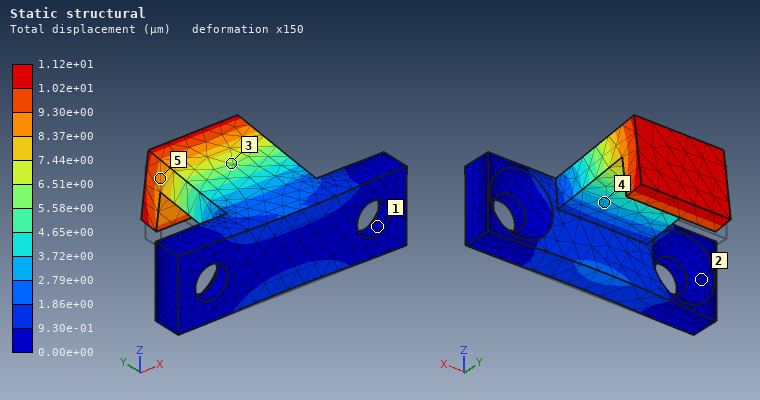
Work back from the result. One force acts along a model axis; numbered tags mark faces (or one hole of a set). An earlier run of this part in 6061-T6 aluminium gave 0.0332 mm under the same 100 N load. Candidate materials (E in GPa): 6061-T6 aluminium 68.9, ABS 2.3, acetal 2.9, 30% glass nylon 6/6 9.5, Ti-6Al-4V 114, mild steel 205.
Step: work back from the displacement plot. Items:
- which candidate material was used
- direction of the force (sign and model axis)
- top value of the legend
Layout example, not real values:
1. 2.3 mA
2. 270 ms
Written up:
1. mild steel
2. +Z
3. 1.12e+01 µm
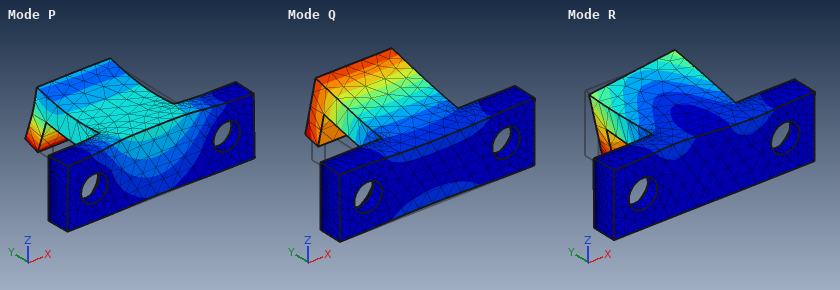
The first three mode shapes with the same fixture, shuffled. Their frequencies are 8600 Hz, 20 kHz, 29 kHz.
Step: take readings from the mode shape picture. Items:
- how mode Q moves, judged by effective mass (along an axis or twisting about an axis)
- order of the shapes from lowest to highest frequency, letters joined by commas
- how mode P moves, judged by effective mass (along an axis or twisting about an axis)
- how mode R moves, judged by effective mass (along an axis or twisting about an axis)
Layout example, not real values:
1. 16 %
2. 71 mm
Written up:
1. along Z
2. Q, R, P
3. along Y
4. along X
